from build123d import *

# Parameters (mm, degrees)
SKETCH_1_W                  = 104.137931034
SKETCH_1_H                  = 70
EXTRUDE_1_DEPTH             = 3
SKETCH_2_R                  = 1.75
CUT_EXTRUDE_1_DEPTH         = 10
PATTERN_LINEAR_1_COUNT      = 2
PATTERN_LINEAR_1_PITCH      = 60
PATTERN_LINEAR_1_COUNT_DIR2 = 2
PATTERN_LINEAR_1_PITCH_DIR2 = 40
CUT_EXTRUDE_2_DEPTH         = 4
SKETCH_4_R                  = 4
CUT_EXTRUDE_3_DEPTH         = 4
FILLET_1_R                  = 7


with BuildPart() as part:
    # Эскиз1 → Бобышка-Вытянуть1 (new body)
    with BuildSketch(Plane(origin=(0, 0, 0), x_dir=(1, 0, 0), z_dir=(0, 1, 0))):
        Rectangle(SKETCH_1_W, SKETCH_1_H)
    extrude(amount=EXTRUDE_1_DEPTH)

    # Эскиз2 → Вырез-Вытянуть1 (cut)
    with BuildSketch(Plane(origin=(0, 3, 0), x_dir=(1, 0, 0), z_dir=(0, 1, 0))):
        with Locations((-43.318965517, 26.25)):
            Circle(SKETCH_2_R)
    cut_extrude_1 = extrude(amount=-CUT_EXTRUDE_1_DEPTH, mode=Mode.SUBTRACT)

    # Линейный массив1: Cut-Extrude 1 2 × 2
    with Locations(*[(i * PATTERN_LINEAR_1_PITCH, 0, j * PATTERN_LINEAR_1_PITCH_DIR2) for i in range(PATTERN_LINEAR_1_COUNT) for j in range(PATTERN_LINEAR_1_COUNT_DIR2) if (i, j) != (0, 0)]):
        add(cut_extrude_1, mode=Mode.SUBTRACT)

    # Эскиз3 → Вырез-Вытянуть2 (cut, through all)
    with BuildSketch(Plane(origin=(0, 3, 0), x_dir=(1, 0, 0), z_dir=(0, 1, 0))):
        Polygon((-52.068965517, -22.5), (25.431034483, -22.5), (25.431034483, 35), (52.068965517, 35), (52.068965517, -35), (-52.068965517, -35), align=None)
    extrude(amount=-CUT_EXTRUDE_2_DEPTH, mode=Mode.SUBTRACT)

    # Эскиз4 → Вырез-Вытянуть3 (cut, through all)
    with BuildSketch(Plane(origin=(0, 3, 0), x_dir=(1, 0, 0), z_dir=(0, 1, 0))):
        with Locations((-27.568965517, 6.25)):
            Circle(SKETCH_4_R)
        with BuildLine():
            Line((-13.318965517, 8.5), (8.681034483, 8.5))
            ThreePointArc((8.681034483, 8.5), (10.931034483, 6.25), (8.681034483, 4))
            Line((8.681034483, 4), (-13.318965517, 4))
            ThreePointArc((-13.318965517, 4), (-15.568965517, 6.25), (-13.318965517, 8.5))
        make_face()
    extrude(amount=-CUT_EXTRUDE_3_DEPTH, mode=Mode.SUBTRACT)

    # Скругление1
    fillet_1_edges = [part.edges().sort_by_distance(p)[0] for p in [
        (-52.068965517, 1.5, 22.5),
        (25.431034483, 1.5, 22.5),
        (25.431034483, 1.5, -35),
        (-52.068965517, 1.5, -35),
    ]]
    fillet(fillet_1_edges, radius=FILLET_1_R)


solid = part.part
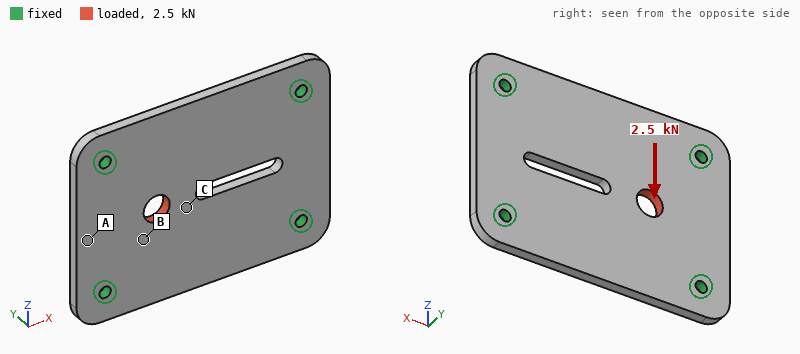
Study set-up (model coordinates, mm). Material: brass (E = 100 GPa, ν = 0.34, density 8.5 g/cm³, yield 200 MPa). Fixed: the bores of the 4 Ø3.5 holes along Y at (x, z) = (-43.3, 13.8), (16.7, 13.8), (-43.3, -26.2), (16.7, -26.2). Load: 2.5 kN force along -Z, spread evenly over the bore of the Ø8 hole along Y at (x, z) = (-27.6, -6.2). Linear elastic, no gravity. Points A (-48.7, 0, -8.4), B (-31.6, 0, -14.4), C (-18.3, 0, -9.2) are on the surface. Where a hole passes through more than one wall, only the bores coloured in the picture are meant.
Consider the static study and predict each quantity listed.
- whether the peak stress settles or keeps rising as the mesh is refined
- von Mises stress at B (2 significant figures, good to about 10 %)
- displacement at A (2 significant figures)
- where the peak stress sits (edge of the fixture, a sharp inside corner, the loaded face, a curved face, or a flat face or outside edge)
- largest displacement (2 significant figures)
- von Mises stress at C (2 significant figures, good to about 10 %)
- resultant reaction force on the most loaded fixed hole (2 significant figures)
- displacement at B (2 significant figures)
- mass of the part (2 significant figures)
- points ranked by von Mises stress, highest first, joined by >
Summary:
keeps rising
28 MPa
1.4 µm
edge of the fixture
8.9 µm
12 MPa
1.0 kN
5.7 µm
110 g
B > C > A
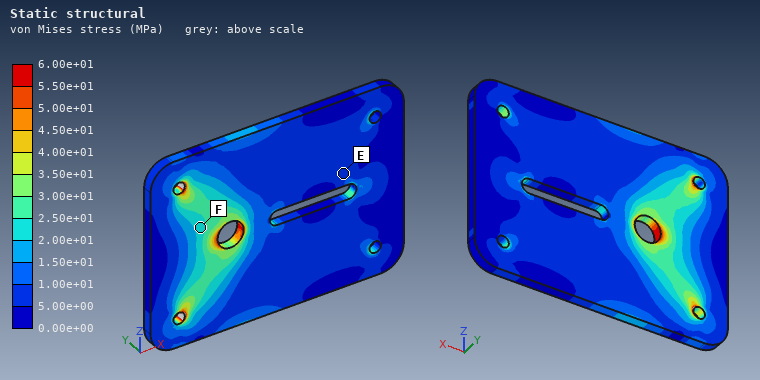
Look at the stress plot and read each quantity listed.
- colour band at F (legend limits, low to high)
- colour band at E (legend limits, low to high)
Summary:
2.00e+01 to 2.50e+01 MPa
5.00e+00 to 1.00e+01 MPa
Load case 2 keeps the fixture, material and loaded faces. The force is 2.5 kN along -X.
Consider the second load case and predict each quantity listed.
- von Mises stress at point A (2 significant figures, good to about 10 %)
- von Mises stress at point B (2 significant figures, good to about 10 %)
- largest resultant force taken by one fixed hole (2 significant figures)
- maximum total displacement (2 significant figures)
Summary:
11 MPa
19 MPa
820 N
7.4 µm
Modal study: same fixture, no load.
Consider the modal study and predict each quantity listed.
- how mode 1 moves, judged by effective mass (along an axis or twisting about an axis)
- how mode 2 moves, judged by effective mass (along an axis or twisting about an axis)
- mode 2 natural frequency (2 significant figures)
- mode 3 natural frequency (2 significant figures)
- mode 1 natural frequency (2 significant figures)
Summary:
along Y
twisting about X
3400 Hz
4500 Hz
2600 Hz
